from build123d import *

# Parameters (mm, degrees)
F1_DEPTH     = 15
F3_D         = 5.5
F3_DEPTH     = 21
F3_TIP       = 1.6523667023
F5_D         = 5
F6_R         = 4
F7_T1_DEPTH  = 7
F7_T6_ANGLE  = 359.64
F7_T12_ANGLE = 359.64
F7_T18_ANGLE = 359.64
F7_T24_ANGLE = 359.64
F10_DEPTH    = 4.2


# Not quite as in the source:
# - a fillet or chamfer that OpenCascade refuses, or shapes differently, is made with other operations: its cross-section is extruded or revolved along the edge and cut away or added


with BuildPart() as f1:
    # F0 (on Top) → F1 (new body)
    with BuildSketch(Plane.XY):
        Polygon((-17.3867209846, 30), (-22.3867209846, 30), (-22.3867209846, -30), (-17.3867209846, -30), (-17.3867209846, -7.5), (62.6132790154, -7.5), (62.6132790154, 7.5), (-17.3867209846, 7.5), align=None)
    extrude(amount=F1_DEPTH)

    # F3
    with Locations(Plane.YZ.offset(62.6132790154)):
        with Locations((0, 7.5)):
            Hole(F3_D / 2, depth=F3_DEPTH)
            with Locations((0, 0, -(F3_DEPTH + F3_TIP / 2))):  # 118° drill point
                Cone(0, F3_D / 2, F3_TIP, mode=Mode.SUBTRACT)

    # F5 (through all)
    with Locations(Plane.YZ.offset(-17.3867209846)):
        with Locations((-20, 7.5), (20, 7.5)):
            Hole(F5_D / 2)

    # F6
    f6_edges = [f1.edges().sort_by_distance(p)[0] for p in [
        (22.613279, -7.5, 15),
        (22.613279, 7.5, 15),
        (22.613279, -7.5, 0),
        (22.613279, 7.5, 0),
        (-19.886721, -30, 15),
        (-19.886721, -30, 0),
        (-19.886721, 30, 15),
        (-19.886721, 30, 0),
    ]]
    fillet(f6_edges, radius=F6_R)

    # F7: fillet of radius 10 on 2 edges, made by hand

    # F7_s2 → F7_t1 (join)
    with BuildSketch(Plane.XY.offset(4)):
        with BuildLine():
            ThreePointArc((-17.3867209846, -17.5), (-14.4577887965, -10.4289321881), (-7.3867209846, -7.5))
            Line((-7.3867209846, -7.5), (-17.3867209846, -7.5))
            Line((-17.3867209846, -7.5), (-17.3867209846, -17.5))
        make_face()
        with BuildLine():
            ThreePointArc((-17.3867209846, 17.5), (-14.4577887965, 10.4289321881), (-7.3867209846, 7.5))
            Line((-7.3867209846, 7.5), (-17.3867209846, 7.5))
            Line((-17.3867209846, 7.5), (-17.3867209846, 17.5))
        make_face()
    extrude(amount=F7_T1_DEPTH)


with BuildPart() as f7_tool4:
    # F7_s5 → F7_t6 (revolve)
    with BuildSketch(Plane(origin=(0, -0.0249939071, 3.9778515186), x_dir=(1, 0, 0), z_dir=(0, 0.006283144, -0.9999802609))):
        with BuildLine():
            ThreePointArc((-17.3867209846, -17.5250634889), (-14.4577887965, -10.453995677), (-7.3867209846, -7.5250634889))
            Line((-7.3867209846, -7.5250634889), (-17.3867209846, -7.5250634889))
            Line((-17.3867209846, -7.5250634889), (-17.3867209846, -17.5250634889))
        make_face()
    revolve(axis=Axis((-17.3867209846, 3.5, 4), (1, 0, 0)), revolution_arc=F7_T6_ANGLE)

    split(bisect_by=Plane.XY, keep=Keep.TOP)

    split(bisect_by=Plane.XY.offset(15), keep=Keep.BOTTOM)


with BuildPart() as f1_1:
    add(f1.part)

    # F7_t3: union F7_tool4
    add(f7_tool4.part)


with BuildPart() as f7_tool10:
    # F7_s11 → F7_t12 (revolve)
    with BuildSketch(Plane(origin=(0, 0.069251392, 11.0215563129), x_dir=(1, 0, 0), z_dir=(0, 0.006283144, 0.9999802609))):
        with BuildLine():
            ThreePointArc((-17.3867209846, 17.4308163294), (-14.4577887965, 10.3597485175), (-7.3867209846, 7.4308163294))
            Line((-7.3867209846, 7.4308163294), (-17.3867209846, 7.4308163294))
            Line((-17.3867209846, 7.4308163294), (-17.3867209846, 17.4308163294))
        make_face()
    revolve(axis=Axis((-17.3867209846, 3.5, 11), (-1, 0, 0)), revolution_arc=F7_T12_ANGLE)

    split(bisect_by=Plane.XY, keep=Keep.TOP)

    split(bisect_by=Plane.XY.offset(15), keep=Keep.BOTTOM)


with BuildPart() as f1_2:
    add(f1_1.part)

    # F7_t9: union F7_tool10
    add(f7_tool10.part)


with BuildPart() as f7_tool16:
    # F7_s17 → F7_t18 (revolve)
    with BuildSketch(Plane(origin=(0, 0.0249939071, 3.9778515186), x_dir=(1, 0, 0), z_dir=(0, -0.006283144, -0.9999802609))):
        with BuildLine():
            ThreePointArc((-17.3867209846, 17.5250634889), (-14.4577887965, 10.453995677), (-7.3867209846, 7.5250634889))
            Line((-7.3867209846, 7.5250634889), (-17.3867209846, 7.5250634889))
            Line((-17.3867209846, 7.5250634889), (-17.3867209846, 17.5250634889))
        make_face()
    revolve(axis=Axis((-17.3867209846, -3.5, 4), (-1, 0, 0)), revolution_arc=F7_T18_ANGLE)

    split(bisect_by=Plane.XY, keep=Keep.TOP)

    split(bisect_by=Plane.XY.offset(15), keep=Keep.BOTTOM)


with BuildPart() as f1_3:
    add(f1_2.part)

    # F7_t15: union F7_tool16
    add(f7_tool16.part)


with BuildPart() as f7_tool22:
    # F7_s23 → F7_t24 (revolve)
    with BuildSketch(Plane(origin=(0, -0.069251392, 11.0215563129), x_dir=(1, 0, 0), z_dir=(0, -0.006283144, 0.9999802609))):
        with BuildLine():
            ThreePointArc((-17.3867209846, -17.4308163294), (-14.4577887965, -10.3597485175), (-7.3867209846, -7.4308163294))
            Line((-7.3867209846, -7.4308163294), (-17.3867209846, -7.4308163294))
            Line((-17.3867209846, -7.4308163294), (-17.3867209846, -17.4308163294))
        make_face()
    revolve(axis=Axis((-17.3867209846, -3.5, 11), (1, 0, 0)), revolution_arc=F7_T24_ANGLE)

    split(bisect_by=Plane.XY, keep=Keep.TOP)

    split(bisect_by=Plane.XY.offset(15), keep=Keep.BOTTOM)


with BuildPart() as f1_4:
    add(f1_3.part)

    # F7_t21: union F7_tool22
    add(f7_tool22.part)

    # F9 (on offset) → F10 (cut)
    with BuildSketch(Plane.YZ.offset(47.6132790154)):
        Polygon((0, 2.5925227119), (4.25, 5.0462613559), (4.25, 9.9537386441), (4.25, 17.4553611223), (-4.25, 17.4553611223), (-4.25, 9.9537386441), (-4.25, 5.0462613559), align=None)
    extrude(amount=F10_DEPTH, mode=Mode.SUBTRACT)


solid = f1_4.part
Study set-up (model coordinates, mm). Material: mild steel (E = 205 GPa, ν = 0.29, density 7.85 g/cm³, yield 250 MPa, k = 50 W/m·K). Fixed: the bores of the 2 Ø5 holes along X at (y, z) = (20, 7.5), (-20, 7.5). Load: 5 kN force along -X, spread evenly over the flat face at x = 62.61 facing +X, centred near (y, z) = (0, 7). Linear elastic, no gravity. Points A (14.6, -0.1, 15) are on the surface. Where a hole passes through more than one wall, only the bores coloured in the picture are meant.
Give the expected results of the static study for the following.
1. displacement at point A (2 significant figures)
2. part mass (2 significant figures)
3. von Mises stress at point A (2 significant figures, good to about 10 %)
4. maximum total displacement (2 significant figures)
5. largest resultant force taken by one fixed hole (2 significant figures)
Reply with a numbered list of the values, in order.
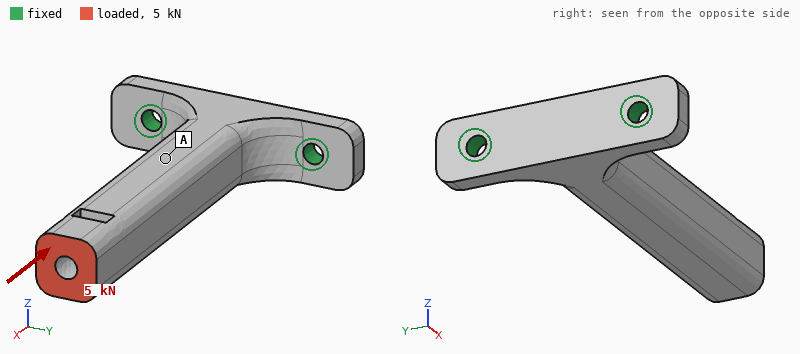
1. 14 µm
2. 160 g
3. 24 MPa
4. 23 µm
5. 3.1 kN
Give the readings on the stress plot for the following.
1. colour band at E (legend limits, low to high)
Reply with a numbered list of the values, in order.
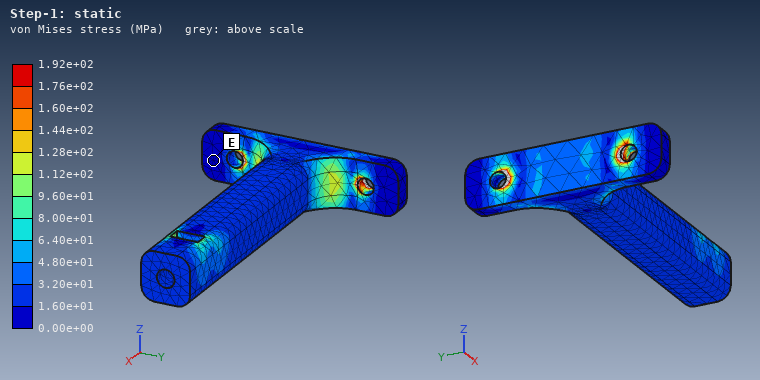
1. 0.00e+00 to 1.60e+01 MPa
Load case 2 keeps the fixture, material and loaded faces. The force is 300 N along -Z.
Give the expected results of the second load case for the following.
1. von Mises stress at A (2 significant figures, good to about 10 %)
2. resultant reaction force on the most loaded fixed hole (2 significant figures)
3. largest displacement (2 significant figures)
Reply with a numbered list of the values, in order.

1. 30 MPa
2. 150 N
3. 0.23 mm
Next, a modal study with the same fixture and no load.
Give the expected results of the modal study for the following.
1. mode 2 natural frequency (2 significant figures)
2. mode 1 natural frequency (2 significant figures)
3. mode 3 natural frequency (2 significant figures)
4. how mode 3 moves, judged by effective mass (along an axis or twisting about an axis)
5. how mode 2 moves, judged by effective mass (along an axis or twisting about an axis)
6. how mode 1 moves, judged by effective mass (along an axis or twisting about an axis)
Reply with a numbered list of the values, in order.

1. 1800 Hz
2. 950 Hz
3. 7400 Hz
4. along Z
5. along Y
6. along Z
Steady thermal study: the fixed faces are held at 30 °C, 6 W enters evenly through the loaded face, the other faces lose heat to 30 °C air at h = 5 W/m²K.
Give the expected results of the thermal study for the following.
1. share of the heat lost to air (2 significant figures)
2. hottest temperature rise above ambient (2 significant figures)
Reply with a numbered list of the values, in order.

1. 12 %
2. 53 K
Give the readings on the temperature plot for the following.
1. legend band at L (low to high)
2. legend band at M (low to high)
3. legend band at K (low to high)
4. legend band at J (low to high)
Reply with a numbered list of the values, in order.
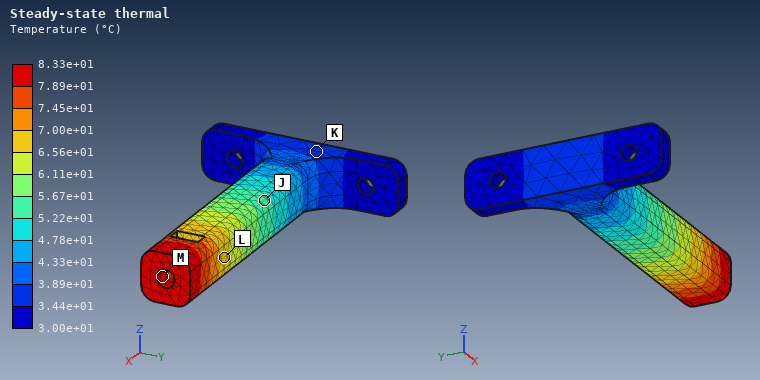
1. 6.56e+01 to 7.00e+01 °C
2. 7.89e+01 to 8.33e+01 °C
3. 3.44e+01 to 3.89e+01 °C
4. 5.22e+01 to 5.67e+01 °C
